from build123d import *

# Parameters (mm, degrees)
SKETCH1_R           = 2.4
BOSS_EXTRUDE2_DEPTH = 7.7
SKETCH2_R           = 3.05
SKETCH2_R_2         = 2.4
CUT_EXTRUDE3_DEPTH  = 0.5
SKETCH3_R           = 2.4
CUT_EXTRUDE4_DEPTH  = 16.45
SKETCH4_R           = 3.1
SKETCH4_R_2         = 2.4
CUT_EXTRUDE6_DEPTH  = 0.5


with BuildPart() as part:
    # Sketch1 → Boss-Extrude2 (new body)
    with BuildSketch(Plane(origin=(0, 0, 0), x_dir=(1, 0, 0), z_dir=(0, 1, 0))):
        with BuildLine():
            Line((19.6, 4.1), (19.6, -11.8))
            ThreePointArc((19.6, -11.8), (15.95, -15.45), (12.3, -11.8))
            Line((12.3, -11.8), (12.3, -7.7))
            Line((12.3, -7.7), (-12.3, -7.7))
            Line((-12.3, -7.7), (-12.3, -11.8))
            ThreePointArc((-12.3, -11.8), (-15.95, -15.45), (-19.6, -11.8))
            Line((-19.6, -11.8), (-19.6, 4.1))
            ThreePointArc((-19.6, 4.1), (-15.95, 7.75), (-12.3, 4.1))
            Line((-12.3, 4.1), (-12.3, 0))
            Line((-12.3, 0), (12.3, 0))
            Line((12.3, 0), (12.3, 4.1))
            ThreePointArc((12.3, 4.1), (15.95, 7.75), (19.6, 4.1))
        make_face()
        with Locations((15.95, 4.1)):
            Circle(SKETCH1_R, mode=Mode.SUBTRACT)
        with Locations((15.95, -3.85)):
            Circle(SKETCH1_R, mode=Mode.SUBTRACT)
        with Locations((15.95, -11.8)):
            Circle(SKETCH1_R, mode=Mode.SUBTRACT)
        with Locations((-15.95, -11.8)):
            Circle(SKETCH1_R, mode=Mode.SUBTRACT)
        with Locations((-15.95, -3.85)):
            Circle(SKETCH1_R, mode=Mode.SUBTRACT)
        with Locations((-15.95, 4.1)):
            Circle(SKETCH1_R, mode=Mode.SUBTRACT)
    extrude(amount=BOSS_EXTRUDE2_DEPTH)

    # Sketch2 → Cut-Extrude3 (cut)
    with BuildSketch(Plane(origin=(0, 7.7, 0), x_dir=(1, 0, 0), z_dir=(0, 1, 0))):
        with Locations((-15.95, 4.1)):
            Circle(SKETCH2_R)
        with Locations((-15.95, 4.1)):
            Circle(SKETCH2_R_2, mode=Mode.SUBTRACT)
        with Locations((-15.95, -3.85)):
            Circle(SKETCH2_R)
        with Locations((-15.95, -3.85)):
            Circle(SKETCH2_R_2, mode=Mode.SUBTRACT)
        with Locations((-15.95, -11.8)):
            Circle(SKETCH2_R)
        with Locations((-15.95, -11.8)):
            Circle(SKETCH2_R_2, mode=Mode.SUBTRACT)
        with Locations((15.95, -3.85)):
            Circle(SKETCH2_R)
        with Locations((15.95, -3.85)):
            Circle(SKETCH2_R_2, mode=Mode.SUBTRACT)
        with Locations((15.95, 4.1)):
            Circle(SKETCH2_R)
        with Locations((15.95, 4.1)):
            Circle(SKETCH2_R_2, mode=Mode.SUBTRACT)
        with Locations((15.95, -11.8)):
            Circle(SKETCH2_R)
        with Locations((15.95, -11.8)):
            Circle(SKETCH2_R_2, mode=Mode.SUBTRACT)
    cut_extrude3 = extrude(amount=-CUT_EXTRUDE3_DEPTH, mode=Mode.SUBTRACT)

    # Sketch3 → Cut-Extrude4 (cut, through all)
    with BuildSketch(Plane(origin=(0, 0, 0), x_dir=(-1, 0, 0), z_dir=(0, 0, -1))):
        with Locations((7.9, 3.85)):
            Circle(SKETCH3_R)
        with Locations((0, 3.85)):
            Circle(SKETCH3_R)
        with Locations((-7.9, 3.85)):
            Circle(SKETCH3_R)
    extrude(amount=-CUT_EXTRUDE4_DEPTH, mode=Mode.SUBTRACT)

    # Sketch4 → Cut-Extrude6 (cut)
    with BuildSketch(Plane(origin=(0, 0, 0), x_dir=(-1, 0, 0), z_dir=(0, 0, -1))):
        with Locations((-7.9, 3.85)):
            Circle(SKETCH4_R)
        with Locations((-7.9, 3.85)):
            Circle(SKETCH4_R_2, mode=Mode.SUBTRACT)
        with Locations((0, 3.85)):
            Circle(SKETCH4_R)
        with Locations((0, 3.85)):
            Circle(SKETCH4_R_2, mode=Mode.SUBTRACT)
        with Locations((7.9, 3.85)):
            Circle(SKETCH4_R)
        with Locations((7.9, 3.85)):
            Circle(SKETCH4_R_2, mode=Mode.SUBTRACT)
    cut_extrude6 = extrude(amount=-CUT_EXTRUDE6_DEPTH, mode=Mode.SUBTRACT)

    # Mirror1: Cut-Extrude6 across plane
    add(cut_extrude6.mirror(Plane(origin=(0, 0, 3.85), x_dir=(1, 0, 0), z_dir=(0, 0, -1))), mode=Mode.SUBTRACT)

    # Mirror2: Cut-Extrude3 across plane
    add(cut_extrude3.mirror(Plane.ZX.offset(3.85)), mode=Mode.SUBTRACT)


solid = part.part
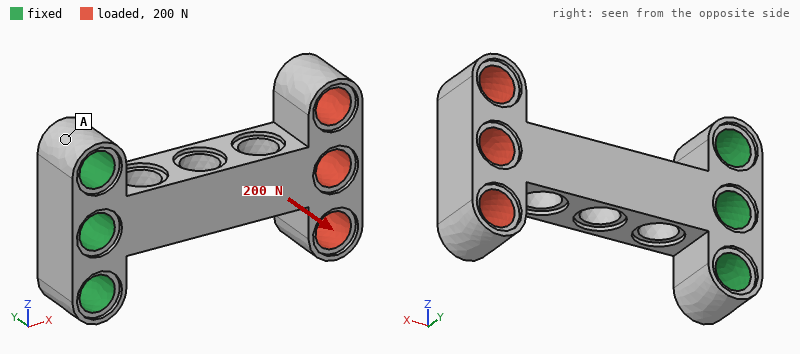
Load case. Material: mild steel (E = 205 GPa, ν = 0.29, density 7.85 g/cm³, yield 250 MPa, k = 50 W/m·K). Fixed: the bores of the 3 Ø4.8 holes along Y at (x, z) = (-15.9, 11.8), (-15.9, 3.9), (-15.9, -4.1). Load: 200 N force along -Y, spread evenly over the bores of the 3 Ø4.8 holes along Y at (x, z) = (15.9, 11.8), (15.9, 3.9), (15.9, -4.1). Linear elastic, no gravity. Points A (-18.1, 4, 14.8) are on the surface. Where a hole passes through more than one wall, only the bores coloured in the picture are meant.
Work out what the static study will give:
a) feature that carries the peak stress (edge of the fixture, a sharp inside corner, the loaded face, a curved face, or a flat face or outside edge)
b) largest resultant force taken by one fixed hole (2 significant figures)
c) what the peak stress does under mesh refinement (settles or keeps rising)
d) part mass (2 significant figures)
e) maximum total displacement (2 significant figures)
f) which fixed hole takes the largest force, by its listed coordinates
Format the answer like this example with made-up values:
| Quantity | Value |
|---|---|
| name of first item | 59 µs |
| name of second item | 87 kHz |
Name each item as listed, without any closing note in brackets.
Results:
| Quantity | Value |
|---|---|
| feature that carries the peak stress | edge of the fixture |
| largest resultant force taken by one fixed hole | 220 N |
| what the peak stress does under mesh refinement | keeps rising |
| part mass | 20 g |
| maximum total displacement | 52 µm |
| which fixed hole takes the largest force, by its listed coordinates | (-15.9, 3.9) |
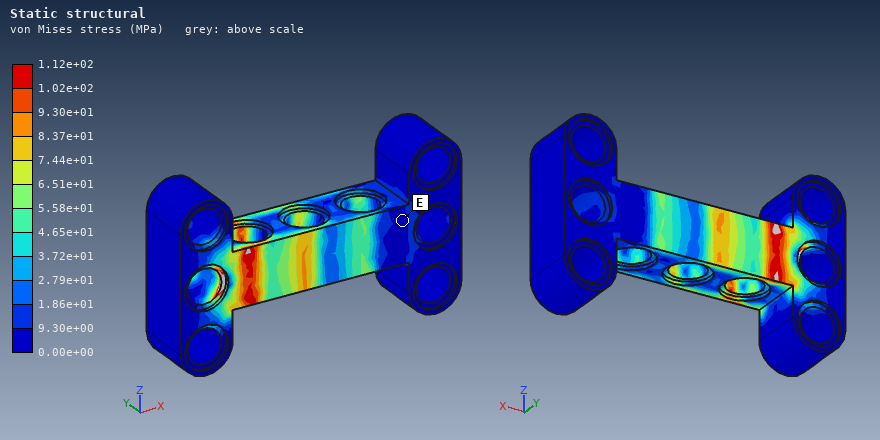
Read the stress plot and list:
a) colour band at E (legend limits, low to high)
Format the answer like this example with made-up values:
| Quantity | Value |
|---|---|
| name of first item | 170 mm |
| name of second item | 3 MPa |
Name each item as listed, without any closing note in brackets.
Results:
| Quantity | Value |
|---|---|
| colour band at E | 0.00e+00 to 9.30e+00 MPa |
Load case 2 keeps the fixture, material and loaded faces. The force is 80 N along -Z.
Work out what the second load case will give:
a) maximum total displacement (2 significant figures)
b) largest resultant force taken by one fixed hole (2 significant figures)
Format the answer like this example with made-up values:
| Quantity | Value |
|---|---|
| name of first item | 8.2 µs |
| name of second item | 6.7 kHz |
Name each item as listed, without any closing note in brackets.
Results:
| Quantity | Value |
|---|---|
| maximum total displacement | 35 µm |
| largest resultant force taken by one fixed hole | 170 N |
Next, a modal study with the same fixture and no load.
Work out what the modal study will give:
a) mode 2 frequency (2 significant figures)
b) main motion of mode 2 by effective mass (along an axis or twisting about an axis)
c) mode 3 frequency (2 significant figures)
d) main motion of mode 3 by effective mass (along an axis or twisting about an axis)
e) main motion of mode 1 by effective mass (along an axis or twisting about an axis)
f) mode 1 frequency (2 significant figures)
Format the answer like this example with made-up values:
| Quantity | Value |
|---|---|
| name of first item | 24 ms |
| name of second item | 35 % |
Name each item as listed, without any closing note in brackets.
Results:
| Quantity | Value |
|---|---|
| mode 2 frequency | 3900 Hz |
| main motion of mode 2 by effective mass | along Y |
| mode 3 frequency | 7400 Hz |
| main motion of mode 3 by effective mass | twisting about X |
| main motion of mode 1 by effective mass | along Z |
| mode 1 frequency | 3100 Hz |
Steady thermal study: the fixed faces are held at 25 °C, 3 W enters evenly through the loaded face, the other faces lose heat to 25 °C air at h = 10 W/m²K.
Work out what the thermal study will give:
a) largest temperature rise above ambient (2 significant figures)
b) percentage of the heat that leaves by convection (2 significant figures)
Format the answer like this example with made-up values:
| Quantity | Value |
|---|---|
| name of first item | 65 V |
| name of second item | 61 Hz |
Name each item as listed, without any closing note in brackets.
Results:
| Quantity | Value |
|---|---|
| largest temperature rise above ambient | 48 K |
| percentage of the heat that leaves by convection | 17 % |
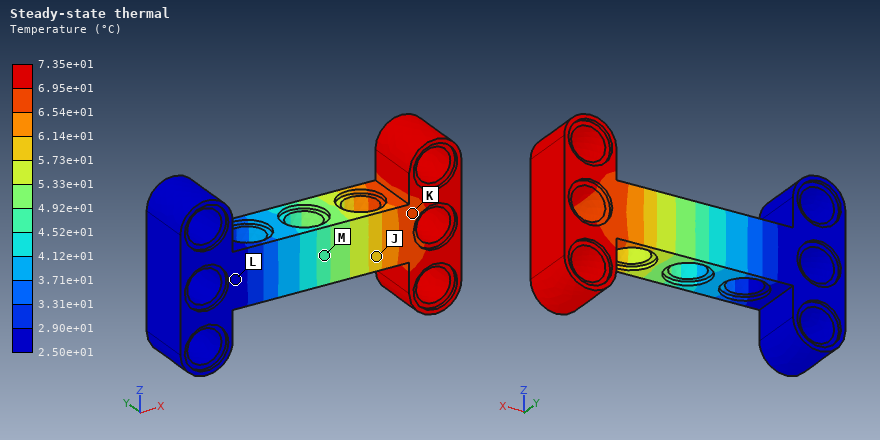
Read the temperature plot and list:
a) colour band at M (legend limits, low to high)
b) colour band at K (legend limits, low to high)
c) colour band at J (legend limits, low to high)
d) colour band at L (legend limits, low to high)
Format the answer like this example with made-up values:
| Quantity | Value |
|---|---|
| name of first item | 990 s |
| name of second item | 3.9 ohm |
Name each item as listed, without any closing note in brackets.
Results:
| Quantity | Value |
|---|---|
| colour band at M | 4.52e+01 to 4.92e+01 °C |
| colour band at K | 6.54e+01 to 6.95e+01 °C |
| colour band at J | 5.73e+01 to 6.14e+01 °C |
| colour band at L | 2.50e+01 to 2.90e+01 °C |
